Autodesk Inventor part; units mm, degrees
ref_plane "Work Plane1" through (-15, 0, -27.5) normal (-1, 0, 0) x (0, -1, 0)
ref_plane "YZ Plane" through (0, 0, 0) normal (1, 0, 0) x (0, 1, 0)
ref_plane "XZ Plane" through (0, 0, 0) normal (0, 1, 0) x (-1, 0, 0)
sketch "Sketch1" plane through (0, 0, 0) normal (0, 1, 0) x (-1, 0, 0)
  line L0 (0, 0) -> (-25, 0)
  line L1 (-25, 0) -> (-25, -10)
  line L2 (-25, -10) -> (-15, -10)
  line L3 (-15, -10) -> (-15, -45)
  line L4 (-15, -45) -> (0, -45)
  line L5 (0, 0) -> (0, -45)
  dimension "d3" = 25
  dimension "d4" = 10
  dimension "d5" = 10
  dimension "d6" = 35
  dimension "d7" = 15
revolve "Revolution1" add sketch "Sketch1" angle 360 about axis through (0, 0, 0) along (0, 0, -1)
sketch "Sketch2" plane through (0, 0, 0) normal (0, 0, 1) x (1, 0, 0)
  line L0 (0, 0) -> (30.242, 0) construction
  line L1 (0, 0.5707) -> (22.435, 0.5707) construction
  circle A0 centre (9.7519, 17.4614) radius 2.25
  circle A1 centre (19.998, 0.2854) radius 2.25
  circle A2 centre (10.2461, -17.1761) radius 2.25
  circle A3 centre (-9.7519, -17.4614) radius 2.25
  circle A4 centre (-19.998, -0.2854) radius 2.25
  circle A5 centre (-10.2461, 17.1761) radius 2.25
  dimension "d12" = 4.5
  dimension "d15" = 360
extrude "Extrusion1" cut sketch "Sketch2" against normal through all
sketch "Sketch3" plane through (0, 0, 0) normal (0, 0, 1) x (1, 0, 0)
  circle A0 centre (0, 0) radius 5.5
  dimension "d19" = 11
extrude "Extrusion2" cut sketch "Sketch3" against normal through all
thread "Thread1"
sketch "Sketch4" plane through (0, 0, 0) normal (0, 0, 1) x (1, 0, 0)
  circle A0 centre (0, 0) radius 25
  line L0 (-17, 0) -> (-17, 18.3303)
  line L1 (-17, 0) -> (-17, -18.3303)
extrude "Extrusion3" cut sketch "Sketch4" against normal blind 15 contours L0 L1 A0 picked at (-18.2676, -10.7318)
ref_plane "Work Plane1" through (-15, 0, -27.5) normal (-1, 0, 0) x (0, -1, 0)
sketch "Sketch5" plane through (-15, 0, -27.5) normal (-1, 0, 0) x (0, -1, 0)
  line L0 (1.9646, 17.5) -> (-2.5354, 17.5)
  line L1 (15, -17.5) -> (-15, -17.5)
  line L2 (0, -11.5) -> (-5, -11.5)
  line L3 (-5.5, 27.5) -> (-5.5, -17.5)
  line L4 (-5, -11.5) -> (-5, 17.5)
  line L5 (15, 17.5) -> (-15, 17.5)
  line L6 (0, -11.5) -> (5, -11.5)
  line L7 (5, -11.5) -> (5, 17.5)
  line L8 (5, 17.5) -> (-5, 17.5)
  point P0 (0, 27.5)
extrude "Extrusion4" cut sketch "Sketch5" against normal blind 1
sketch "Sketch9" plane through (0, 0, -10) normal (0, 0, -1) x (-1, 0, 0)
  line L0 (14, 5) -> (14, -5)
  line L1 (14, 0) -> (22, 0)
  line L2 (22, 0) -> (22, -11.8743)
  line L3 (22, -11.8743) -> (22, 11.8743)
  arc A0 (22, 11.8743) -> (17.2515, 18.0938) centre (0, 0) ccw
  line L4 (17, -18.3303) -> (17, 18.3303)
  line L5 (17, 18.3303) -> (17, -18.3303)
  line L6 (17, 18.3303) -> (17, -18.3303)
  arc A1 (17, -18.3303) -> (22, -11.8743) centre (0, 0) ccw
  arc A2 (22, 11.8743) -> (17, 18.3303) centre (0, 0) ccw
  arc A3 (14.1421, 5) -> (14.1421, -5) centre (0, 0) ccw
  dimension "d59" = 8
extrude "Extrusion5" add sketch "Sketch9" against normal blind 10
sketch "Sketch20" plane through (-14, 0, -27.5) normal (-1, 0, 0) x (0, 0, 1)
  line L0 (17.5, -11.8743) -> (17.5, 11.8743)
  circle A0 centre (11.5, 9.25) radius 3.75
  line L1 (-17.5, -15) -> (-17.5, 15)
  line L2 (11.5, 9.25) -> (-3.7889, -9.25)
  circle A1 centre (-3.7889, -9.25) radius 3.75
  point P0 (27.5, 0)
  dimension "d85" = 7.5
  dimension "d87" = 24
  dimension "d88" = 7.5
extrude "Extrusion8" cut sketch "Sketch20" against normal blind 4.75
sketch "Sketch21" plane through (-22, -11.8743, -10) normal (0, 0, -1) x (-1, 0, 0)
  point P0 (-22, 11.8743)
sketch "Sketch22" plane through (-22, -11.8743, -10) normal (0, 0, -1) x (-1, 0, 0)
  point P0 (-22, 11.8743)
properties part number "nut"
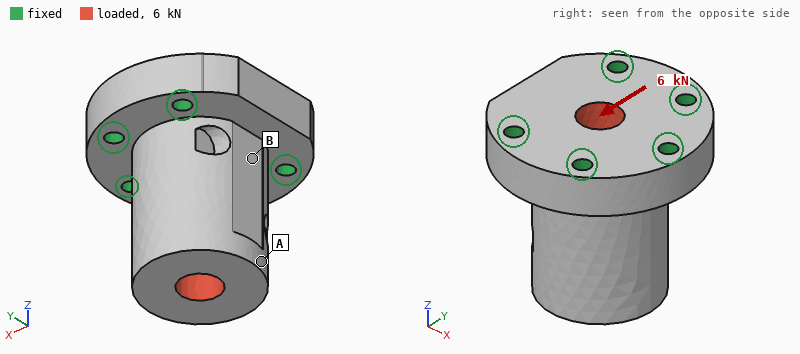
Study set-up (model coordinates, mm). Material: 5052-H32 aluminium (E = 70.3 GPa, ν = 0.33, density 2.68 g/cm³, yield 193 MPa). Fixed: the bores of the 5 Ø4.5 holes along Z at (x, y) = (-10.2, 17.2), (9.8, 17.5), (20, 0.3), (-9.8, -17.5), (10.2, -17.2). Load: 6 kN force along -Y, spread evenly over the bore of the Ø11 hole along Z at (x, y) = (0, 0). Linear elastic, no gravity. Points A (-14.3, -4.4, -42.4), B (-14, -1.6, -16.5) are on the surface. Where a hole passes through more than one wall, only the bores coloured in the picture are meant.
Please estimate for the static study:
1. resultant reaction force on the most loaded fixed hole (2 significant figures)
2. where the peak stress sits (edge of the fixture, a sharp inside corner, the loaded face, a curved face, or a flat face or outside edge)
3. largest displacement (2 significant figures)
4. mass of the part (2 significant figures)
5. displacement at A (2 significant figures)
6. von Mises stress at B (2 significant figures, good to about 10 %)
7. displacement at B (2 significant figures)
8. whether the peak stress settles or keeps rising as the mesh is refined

2.3 kN
edge of the fixture
30 µm
100 g
26 µm
15 MPa
6.2 µm
keeps rising
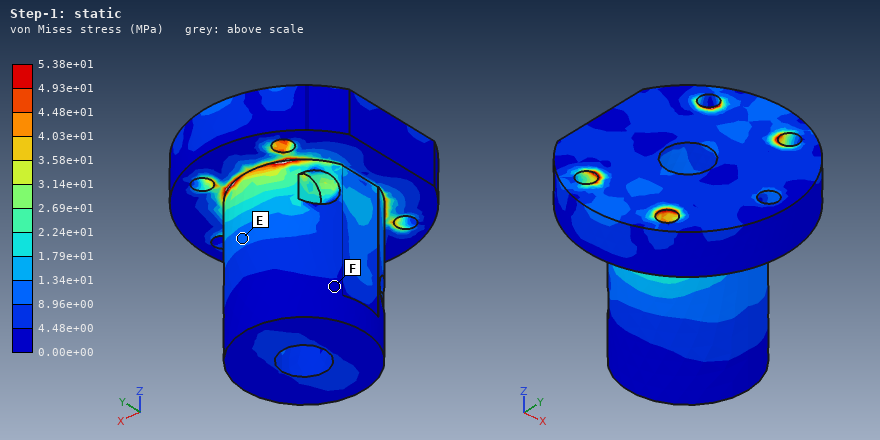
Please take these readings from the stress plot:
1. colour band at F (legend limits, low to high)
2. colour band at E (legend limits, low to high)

0.00e+00 to 4.48e+00 MPa
8.96e+00 to 1.34e+01 MPa
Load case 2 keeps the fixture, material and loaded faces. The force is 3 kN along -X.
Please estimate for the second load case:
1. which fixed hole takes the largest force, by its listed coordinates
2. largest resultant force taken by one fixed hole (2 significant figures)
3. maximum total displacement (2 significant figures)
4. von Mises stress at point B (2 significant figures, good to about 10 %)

(20, 0.3)
1.4 kN
19 µm
8.1 MPa
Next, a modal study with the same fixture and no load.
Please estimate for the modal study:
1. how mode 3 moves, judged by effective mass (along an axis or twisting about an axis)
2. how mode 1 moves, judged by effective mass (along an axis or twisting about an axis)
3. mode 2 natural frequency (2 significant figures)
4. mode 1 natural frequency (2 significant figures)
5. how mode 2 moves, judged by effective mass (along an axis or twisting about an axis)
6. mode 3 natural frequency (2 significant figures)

twisting about Z
along X
10 kHz
8800 Hz
along Y
20 kHz
